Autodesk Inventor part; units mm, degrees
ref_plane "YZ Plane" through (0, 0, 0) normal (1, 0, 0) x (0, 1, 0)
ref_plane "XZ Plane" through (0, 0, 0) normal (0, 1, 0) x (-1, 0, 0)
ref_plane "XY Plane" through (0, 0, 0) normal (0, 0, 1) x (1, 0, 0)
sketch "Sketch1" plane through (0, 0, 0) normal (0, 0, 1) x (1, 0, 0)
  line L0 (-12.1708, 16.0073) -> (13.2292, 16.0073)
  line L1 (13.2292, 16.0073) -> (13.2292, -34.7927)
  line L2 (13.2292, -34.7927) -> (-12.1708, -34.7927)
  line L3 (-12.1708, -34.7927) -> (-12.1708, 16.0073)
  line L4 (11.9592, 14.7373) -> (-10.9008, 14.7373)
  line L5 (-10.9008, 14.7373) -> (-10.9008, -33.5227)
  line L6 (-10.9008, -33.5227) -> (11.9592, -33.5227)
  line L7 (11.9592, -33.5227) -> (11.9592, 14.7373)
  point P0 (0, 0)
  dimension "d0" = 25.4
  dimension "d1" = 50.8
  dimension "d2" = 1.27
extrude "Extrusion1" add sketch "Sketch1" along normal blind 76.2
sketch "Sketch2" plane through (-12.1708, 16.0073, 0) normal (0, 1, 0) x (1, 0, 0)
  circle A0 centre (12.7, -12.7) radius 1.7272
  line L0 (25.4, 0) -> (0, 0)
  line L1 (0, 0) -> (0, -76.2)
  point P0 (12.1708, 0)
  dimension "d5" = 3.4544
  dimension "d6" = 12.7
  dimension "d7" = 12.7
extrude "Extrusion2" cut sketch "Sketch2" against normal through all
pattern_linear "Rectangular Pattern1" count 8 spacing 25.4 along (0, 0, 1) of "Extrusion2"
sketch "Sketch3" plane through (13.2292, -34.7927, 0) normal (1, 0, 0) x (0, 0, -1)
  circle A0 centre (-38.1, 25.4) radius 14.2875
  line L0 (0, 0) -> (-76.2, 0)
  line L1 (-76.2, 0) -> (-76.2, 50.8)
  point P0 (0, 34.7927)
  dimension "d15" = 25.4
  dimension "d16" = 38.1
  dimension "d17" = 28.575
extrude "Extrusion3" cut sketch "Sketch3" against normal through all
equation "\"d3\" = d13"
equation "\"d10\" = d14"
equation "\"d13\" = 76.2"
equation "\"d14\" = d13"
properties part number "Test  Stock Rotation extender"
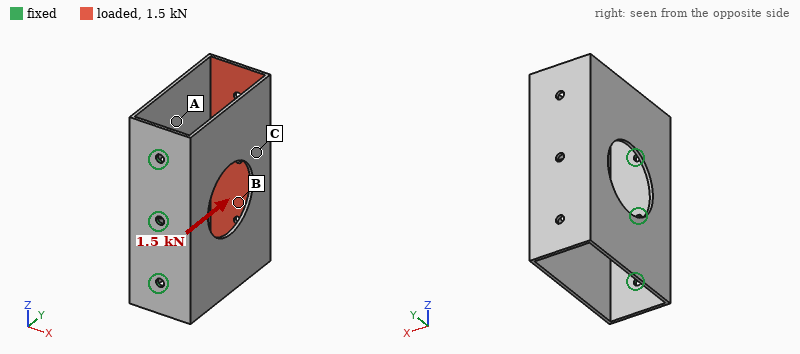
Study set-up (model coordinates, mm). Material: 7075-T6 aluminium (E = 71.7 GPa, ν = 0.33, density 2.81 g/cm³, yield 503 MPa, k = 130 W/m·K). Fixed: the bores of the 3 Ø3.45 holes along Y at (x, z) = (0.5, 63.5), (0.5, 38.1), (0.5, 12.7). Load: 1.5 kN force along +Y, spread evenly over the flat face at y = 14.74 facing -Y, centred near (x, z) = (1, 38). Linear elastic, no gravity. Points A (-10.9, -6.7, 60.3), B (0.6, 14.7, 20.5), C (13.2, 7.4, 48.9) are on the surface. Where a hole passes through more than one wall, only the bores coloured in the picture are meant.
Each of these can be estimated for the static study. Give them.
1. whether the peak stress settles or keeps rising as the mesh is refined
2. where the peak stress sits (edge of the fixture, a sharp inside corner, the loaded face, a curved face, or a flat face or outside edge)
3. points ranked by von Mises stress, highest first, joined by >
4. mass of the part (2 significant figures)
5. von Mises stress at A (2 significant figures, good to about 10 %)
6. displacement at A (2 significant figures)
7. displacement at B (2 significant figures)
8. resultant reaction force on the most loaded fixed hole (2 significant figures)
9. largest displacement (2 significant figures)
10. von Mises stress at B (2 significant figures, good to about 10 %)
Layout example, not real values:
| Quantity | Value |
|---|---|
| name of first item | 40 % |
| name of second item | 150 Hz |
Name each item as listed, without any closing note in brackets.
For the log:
| Quantity | Value |
|---|---|
| whether the peak stress settles or keeps rising as the mesh is refined | keeps rising |
| where the peak stress sits | edge of the fixture |
| points ranked by von Mises stress, highest first, joined by > | B > A > C |
| mass of the part | 35 g |
| von Mises stress at A | 85 MPa |
| displacement at A | 0.54 mm |
| displacement at B | 0.57 mm |
| resultant reaction force on the most loaded fixed hole | 520 N |
| largest displacement | 0.59 mm |
| von Mises stress at B | 190 MPa |
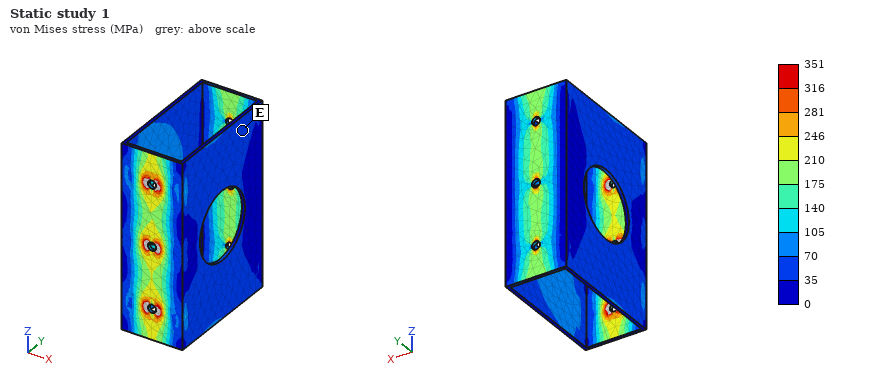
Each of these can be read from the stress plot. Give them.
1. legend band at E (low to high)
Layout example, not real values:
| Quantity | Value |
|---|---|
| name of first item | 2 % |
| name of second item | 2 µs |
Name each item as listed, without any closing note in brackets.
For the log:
| Quantity | Value |
|---|---|
| legend band at E | 35 to 70 MPa |
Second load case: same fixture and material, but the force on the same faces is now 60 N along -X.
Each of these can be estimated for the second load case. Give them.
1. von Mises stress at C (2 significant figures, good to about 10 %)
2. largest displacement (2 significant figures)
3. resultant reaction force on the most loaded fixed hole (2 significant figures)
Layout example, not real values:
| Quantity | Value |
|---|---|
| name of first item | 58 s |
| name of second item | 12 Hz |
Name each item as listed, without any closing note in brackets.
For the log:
| Quantity | Value |
|---|---|
| von Mises stress at C | 25 MPa |
| largest displacement | 1.0 mm |
| resultant reaction force on the most loaded fixed hole | 25 N |
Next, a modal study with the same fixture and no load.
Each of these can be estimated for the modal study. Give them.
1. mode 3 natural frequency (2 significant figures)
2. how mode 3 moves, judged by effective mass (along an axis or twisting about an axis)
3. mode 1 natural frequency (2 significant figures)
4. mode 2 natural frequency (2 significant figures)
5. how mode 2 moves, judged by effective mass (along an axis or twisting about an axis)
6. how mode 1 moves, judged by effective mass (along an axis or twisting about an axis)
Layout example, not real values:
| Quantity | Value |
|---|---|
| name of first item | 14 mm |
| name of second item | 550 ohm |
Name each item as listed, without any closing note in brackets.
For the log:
| Quantity | Value |
|---|---|
| mode 3 natural frequency | 1100 Hz |
| how mode 3 moves, judged by effective mass | along Z |
| mode 1 natural frequency | 320 Hz |
| mode 2 natural frequency | 1100 Hz |
| how mode 2 moves, judged by effective mass | twisting about Y |
| how mode 1 moves, judged by effective mass | along X |
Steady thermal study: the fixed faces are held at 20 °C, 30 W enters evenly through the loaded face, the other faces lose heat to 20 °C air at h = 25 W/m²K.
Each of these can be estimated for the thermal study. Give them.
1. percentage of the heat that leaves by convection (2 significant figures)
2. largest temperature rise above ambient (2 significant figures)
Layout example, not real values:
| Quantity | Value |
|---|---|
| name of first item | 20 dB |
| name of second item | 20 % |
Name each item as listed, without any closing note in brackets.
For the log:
| Quantity | Value |
|---|---|
| percentage of the heat that leaves by convection | 51 % |
| largest temperature rise above ambient | 70 K |
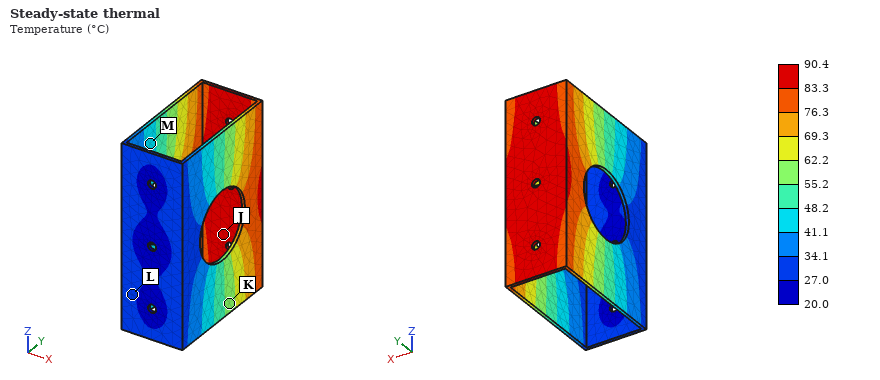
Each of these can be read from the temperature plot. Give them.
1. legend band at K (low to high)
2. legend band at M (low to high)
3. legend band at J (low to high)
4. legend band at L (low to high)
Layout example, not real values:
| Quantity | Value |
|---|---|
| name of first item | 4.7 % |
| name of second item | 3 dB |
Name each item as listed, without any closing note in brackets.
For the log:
| Quantity | Value |
|---|---|
| legend band at K | 55.2 to 62.2 °C |
| legend band at M | 41.1 to 48.2 °C |
| legend band at J | 83.3 to 90.4 °C |
| legend band at L | 27.0 to 34.1 °C |
